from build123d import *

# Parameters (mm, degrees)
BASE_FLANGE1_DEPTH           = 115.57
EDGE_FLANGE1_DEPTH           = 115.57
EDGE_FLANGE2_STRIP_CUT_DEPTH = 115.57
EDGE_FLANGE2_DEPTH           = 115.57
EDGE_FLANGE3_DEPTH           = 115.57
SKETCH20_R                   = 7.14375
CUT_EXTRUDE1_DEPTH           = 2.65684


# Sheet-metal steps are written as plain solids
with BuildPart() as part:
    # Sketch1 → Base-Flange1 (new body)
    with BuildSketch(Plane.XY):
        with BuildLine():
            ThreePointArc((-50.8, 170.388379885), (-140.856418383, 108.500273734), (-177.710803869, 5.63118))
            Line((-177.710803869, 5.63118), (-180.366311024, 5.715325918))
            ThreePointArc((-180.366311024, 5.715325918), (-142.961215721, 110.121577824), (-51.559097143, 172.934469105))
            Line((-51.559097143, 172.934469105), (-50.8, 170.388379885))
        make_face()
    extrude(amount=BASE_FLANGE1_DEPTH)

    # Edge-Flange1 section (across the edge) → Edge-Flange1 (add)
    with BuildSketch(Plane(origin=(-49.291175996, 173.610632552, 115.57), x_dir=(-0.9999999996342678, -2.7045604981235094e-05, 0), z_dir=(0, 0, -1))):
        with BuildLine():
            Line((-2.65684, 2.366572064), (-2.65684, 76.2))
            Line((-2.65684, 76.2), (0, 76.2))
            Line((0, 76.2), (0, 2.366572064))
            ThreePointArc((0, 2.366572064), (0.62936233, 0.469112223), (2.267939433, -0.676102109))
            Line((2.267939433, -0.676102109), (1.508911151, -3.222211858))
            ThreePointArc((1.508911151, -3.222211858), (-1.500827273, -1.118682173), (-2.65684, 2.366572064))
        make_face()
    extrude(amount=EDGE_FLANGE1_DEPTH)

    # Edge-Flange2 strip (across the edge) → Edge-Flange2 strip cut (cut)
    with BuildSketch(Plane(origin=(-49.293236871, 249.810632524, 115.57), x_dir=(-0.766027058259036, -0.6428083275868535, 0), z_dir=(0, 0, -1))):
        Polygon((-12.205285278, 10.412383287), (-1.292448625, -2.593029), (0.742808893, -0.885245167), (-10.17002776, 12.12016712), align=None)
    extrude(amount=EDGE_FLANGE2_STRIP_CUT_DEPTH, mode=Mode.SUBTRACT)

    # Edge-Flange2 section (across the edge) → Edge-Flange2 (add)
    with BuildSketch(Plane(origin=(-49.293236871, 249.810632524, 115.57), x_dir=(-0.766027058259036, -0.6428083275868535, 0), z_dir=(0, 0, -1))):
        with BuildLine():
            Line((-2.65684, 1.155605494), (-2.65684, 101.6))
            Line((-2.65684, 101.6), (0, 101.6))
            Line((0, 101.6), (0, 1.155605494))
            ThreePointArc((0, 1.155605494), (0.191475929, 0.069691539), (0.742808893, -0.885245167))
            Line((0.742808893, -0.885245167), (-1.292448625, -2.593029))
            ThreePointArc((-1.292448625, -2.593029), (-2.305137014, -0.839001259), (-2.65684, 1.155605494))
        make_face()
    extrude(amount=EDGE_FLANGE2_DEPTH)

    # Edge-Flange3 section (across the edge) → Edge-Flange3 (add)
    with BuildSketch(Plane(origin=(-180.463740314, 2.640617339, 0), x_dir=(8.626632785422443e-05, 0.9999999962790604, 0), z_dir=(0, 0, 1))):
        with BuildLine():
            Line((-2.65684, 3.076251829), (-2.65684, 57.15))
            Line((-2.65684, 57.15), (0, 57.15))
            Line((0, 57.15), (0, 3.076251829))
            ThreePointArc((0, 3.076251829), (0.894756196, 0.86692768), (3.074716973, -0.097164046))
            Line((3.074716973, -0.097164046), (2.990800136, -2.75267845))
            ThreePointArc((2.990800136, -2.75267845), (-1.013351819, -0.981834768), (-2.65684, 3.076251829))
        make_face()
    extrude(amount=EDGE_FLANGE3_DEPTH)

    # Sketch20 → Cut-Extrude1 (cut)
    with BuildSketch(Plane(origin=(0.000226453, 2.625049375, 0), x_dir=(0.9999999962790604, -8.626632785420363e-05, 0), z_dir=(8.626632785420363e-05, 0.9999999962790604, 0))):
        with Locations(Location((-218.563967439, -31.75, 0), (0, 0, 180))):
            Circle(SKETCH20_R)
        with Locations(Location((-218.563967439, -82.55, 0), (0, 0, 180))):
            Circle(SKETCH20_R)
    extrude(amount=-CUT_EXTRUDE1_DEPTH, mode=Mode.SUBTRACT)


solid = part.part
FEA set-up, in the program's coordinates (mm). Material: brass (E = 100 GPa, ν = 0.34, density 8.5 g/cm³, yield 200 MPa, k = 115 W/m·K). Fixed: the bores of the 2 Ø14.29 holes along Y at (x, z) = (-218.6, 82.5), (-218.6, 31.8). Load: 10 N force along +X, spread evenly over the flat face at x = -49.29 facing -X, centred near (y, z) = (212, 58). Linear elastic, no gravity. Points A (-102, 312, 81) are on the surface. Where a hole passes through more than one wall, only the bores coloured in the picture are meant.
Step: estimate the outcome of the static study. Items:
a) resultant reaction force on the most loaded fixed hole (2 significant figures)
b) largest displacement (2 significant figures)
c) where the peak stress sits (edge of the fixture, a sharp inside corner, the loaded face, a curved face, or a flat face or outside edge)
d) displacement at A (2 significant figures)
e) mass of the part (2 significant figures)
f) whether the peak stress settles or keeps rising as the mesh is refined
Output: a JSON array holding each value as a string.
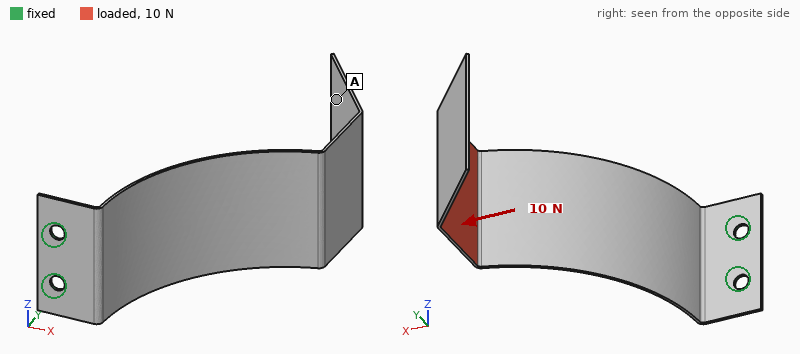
["6.4 N", "4.6 mm", "edge of the fixture", "4.3 mm", "1.2 kg", "keeps rising"]
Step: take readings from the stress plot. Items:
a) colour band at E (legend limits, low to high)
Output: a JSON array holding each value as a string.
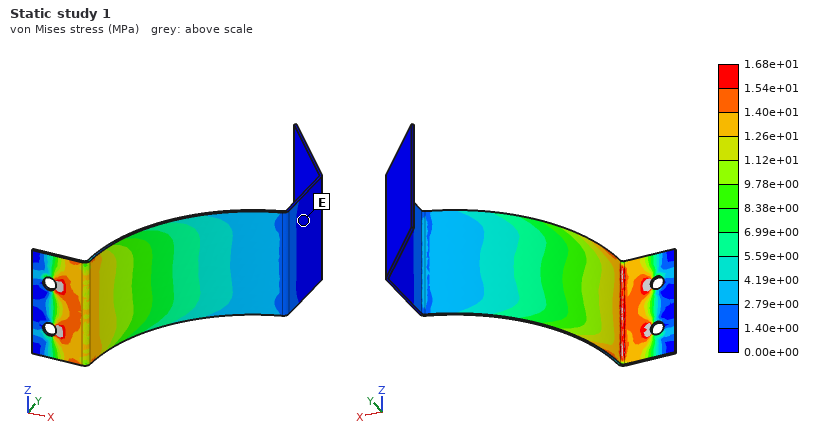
["0.00e+00 to 1.40e+00 MPa"]
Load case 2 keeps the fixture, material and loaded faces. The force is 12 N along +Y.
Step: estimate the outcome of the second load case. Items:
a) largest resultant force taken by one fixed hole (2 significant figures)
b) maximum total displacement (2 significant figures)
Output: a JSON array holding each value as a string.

["6.8 N", "4.0 mm"]
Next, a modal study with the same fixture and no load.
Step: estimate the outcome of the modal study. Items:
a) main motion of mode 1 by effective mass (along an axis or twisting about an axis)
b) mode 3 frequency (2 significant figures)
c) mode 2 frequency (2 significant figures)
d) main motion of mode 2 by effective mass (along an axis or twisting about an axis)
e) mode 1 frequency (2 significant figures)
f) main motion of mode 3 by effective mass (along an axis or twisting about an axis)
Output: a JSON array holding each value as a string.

["along X", "45 Hz", "32 Hz", "along Z", "9.1 Hz", "along Y"]
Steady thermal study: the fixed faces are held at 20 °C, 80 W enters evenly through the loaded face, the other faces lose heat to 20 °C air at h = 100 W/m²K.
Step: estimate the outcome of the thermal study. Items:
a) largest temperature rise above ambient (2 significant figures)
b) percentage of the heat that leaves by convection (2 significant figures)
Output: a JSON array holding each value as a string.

["39 K", "100 %"]
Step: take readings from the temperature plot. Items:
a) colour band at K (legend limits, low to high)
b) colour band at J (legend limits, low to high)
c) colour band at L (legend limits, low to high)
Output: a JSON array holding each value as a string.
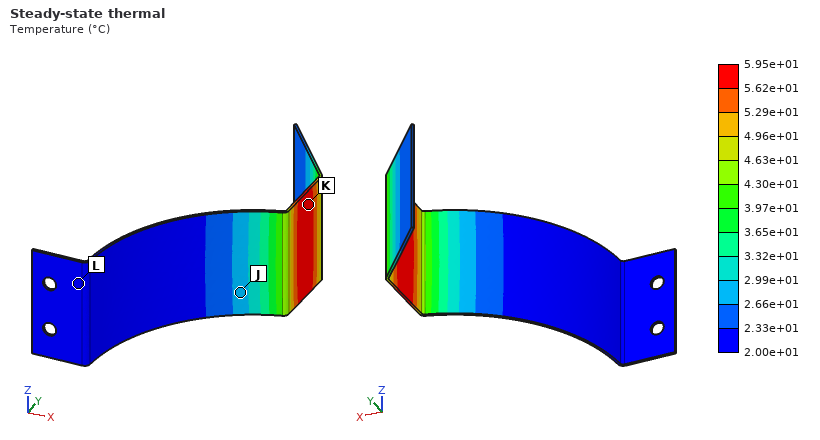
["5.62e+01 to 5.95e+01 °C", "2.66e+01 to 2.99e+01 °C", "2.00e+01 to 2.33e+01 °C"]
